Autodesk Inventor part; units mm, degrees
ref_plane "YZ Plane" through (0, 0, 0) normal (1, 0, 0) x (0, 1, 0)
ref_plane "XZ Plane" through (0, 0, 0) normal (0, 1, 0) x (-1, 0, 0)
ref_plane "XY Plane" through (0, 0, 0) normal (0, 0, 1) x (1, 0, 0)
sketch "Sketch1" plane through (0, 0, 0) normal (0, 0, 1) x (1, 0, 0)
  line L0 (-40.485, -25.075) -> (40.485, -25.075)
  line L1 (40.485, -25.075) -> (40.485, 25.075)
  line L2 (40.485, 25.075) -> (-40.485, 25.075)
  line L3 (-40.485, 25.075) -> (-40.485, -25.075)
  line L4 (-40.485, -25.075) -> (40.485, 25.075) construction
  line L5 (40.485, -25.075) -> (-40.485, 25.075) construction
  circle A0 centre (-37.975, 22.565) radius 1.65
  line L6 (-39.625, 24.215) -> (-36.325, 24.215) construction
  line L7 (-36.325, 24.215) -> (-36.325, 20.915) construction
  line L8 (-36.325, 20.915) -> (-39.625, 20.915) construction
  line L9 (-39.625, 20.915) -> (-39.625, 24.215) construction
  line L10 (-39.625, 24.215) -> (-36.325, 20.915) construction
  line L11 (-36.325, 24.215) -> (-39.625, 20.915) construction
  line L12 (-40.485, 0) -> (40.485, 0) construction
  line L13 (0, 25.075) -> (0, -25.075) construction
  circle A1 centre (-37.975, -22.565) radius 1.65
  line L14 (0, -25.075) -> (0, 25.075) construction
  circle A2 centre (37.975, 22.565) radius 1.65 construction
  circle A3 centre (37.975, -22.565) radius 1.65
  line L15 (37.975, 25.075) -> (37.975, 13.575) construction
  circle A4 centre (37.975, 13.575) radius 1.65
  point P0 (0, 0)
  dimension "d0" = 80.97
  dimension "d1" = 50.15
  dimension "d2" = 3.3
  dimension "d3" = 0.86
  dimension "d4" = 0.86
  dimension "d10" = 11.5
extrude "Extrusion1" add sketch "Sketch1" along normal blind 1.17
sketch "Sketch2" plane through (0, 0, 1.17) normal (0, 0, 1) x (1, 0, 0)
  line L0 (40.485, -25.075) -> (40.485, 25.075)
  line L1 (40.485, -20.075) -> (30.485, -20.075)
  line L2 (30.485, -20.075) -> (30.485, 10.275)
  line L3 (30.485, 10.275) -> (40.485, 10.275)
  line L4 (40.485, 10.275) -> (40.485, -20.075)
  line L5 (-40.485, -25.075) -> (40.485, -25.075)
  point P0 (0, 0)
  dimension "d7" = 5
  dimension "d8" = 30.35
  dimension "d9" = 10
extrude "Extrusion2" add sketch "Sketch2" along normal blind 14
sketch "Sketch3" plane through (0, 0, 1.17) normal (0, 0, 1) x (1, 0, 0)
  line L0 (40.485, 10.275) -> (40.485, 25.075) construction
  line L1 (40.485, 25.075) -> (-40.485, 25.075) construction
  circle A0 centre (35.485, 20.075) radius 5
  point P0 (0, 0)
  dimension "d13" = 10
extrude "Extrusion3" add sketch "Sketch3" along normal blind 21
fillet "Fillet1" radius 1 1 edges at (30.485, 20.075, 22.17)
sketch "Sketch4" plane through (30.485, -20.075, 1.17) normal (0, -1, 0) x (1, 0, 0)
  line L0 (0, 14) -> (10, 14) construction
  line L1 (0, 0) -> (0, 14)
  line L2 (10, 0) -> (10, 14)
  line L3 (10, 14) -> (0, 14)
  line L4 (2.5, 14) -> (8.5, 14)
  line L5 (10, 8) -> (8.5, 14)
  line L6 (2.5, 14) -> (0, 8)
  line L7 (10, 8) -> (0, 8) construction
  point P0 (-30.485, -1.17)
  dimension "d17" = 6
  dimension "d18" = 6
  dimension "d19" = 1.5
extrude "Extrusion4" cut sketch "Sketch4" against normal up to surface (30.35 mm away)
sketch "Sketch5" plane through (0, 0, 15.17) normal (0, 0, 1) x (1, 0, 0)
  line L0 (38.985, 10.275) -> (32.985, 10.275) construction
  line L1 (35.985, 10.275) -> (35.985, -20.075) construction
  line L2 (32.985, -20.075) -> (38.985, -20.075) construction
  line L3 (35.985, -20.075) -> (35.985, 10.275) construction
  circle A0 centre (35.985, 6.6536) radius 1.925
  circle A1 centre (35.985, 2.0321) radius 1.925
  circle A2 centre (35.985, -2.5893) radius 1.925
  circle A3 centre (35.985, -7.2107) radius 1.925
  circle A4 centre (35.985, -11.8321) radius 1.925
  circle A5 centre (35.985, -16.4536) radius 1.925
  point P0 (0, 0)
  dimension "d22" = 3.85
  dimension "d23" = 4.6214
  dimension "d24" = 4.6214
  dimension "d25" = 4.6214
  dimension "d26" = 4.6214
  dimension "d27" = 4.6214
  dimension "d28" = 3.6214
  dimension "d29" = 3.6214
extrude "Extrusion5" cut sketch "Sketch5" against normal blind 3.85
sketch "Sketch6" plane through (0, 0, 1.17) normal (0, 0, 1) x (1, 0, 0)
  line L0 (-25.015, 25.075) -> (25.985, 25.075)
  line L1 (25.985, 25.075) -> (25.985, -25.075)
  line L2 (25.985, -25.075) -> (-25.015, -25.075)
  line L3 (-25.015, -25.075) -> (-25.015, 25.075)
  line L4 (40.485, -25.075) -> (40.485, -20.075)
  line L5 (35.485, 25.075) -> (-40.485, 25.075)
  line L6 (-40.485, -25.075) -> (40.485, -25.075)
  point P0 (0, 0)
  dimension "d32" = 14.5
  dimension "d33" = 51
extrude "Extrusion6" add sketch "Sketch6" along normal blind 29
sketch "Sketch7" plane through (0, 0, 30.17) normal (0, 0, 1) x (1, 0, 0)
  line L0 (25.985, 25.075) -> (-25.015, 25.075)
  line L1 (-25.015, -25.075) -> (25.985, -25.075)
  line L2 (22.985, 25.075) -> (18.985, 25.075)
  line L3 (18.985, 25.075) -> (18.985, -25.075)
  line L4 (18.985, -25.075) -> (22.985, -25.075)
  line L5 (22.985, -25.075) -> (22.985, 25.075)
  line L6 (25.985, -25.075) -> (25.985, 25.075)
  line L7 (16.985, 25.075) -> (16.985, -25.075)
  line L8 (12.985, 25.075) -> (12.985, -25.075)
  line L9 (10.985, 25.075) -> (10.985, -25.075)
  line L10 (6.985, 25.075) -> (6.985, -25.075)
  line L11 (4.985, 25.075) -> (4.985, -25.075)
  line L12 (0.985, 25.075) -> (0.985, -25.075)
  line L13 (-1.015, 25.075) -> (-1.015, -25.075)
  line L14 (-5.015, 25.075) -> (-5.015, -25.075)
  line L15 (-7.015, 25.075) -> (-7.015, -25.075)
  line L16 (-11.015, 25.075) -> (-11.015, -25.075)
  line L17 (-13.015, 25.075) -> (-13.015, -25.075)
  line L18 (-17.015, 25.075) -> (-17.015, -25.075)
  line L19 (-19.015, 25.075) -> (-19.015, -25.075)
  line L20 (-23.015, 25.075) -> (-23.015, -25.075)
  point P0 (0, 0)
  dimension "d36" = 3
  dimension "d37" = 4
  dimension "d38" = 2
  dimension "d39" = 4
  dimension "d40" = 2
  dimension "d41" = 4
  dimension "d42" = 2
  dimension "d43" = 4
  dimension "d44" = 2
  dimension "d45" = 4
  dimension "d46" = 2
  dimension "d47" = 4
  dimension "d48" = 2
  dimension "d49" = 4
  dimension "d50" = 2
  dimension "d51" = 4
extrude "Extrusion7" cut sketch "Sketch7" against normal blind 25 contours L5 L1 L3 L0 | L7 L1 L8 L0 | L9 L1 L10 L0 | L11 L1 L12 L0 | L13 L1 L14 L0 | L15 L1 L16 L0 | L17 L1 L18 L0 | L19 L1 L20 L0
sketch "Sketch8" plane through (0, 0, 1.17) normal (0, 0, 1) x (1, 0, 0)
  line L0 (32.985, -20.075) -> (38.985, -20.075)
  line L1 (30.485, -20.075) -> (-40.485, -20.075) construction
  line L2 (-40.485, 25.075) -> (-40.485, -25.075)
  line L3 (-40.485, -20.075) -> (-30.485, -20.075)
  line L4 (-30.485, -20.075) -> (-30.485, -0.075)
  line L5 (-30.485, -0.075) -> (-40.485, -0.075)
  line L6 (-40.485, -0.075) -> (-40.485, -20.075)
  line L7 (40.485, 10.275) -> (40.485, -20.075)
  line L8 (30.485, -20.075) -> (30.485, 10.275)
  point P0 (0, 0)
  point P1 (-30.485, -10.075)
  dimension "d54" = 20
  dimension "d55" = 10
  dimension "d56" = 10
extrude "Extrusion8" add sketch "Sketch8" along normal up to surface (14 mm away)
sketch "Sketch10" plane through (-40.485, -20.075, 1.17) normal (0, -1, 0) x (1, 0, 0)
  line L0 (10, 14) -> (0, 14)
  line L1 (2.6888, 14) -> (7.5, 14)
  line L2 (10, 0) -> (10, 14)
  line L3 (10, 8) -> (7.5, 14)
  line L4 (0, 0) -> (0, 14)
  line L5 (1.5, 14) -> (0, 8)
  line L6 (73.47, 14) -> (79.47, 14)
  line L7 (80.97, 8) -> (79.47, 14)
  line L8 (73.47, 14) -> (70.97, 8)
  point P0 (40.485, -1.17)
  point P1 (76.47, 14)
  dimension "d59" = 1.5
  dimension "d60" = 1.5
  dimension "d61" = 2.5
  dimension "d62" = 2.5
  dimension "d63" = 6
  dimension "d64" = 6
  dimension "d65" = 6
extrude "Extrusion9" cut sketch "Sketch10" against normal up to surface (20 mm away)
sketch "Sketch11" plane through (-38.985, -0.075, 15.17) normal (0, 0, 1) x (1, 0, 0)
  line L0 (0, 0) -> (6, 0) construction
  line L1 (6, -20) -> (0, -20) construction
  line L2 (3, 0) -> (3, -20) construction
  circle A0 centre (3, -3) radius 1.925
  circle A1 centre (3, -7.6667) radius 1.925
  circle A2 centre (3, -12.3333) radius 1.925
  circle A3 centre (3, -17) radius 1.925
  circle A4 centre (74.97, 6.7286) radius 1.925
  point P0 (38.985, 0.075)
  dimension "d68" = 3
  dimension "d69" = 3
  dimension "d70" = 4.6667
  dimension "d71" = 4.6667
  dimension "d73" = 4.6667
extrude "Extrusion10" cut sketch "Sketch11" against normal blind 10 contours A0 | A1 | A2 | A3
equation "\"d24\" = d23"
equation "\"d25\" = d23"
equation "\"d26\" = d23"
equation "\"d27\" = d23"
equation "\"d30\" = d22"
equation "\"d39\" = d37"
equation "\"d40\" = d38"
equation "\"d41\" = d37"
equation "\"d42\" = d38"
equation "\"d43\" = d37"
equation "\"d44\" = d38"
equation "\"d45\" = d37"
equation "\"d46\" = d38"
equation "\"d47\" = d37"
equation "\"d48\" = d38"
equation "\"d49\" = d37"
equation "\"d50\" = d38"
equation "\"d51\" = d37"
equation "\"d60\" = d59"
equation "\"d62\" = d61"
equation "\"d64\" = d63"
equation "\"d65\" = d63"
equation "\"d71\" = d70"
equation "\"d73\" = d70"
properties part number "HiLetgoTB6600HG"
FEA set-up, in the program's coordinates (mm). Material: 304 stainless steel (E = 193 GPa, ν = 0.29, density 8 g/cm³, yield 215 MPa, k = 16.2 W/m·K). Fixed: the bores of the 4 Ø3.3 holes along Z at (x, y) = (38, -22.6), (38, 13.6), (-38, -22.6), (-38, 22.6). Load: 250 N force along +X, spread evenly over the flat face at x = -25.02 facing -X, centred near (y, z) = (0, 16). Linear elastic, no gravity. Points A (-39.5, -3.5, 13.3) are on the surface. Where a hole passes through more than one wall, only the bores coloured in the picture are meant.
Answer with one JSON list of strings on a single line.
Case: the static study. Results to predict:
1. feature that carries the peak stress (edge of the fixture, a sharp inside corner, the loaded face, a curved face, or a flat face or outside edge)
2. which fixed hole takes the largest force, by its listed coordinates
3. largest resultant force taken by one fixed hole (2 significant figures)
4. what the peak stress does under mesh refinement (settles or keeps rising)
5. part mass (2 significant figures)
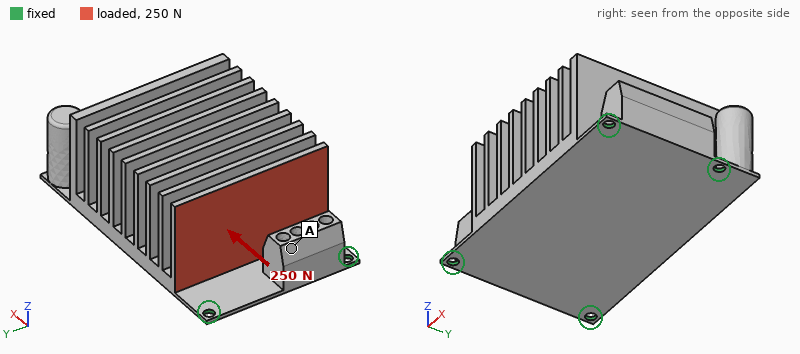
["edge of the fixture", "(38, 13.6)", "150 N", "keeps rising", "370 g"]
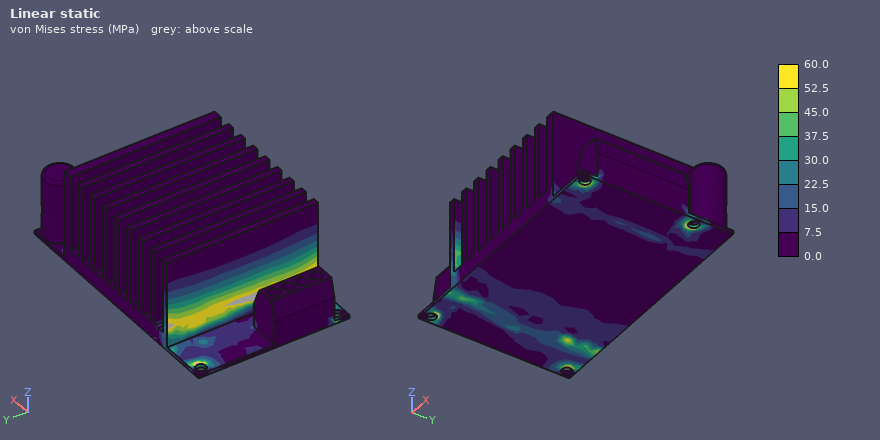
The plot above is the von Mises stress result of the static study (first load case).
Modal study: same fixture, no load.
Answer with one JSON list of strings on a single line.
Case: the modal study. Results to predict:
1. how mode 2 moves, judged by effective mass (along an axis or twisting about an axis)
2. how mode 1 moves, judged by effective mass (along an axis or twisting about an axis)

["along Y", "along Z"]
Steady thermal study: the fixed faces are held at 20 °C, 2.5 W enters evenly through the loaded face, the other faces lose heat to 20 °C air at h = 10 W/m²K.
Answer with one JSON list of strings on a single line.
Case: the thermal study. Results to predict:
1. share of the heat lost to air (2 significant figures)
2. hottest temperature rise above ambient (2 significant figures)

["75 %", "27 K"]
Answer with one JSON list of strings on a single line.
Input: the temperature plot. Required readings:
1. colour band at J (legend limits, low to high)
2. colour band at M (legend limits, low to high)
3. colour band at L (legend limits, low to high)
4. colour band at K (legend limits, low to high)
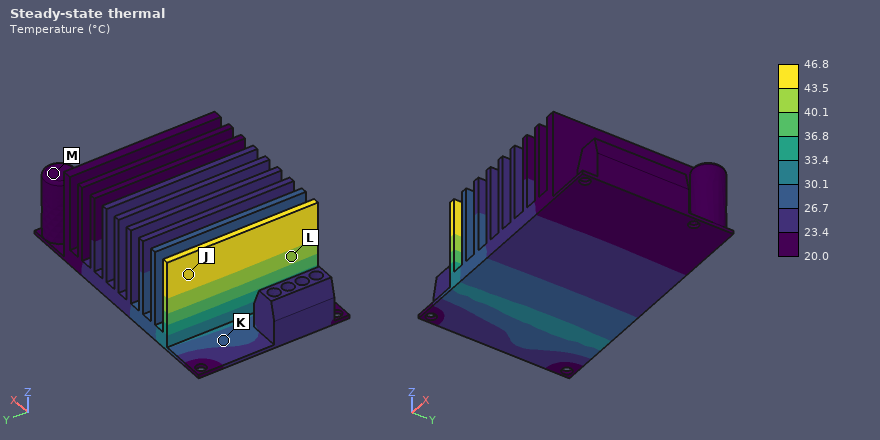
["43.5 to 46.8 °C", "20.0 to 23.4 °C", "40.1 to 43.5 °C", "26.7 to 30.1 °C"]
